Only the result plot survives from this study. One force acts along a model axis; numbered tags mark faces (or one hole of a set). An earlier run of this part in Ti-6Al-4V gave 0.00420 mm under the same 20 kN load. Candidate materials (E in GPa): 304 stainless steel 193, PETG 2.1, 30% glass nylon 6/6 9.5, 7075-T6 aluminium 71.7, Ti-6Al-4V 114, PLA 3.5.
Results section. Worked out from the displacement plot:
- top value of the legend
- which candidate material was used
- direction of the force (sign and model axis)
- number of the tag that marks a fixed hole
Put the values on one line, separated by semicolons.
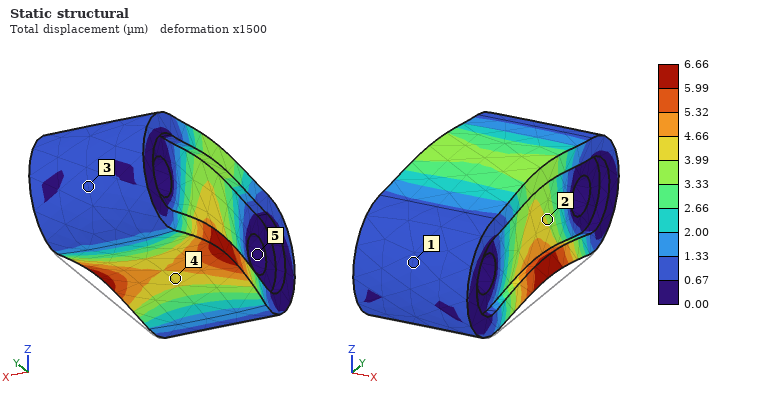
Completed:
6.66 µm; 7075-T6 aluminium; +Z; 5
